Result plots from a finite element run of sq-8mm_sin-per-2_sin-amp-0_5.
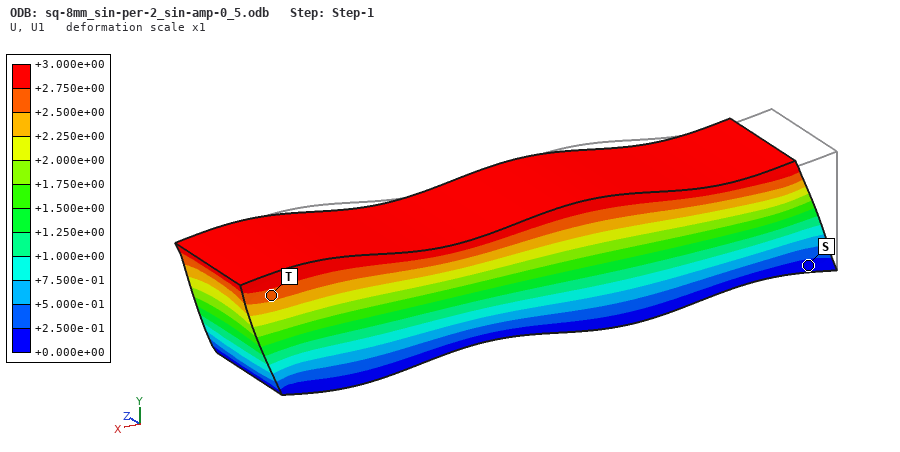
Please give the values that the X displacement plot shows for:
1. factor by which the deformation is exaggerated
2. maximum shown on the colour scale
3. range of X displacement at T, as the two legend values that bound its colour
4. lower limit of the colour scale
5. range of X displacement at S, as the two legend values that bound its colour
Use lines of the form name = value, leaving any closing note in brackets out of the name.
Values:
factor by which the deformation is exaggerated = 1
maximum shown on the colour scale = +3.000e+00
range of X displacement at T, as the two legend values that bound its colour = +2.500e+00 to +2.750e+00
lower limit of the colour scale = +0.000e+00
range of X displacement at S, as the two legend values that bound its colour = +0.000e+00 to +2.500e-01
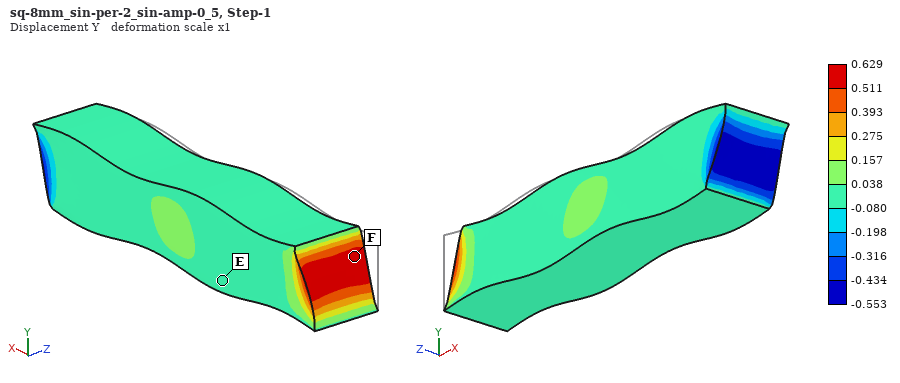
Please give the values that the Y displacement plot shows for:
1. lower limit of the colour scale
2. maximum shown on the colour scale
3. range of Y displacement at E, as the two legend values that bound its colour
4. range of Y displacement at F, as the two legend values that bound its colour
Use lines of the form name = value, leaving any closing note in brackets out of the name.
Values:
lower limit of the colour scale = -0.553
maximum shown on the colour scale = 0.629
range of Y displacement at E, as the two legend values that bound its colour = -0.080 to 0.038
range of Y displacement at F, as the two legend values that bound its colour = 0.511 to 0.629
